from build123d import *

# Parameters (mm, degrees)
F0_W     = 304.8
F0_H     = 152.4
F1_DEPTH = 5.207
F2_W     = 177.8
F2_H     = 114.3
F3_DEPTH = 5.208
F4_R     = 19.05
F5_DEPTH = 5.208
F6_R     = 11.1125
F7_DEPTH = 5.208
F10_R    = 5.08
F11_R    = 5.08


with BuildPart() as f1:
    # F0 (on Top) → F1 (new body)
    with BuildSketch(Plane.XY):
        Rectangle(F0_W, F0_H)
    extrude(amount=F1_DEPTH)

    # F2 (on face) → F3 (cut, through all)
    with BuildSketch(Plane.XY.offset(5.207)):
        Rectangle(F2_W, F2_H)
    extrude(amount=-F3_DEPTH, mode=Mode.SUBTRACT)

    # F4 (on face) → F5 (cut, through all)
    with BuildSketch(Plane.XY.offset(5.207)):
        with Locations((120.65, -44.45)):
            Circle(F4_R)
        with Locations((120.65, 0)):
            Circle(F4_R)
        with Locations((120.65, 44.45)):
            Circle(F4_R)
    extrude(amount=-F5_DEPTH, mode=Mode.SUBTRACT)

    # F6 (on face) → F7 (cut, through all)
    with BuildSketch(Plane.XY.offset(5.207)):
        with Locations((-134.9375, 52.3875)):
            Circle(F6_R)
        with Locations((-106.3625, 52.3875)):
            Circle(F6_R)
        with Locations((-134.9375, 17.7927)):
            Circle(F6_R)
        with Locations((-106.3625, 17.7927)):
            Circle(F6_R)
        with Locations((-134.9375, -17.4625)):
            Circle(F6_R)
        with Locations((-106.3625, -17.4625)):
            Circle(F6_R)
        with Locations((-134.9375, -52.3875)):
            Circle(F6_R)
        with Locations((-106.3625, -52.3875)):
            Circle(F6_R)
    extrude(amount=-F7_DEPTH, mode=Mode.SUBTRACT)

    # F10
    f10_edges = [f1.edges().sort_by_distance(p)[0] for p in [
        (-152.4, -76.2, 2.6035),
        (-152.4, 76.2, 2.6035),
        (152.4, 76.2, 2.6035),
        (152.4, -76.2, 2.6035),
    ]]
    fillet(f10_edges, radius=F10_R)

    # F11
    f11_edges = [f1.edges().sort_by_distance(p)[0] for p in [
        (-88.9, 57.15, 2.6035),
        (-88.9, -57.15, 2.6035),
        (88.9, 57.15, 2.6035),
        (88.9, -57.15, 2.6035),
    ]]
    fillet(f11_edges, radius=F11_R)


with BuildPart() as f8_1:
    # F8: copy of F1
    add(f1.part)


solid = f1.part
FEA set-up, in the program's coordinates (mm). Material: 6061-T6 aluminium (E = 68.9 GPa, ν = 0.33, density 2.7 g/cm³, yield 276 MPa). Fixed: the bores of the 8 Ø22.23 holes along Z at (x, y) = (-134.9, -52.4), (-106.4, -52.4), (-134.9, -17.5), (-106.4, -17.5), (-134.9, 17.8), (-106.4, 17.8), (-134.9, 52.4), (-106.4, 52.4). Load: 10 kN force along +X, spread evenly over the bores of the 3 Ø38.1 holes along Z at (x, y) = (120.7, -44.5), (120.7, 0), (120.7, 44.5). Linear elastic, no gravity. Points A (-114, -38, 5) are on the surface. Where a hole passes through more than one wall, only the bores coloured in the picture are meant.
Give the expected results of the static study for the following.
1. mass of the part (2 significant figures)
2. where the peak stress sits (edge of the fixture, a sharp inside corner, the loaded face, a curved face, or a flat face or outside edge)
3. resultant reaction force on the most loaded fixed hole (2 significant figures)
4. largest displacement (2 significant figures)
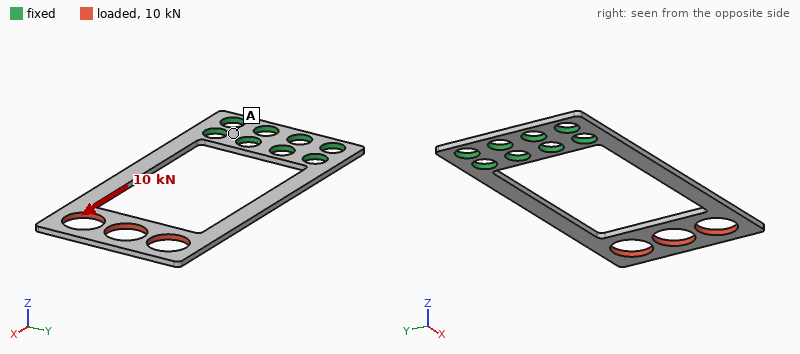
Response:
280 g
the loaded face
4.3 kN
0.38 mm
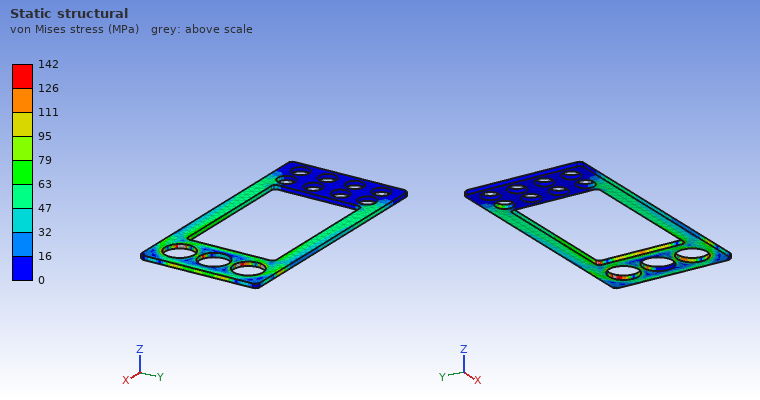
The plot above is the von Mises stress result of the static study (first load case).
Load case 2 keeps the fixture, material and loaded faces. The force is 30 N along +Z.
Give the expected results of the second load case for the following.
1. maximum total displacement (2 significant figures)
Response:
4.1 mm
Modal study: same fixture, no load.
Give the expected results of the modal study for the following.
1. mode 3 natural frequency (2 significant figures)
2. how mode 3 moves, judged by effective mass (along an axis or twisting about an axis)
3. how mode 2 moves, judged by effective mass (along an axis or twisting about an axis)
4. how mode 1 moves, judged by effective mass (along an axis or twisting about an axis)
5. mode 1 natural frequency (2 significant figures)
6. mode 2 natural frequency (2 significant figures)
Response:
350 Hz
along Y
twisting about X
along Z
47 Hz
160 Hz
